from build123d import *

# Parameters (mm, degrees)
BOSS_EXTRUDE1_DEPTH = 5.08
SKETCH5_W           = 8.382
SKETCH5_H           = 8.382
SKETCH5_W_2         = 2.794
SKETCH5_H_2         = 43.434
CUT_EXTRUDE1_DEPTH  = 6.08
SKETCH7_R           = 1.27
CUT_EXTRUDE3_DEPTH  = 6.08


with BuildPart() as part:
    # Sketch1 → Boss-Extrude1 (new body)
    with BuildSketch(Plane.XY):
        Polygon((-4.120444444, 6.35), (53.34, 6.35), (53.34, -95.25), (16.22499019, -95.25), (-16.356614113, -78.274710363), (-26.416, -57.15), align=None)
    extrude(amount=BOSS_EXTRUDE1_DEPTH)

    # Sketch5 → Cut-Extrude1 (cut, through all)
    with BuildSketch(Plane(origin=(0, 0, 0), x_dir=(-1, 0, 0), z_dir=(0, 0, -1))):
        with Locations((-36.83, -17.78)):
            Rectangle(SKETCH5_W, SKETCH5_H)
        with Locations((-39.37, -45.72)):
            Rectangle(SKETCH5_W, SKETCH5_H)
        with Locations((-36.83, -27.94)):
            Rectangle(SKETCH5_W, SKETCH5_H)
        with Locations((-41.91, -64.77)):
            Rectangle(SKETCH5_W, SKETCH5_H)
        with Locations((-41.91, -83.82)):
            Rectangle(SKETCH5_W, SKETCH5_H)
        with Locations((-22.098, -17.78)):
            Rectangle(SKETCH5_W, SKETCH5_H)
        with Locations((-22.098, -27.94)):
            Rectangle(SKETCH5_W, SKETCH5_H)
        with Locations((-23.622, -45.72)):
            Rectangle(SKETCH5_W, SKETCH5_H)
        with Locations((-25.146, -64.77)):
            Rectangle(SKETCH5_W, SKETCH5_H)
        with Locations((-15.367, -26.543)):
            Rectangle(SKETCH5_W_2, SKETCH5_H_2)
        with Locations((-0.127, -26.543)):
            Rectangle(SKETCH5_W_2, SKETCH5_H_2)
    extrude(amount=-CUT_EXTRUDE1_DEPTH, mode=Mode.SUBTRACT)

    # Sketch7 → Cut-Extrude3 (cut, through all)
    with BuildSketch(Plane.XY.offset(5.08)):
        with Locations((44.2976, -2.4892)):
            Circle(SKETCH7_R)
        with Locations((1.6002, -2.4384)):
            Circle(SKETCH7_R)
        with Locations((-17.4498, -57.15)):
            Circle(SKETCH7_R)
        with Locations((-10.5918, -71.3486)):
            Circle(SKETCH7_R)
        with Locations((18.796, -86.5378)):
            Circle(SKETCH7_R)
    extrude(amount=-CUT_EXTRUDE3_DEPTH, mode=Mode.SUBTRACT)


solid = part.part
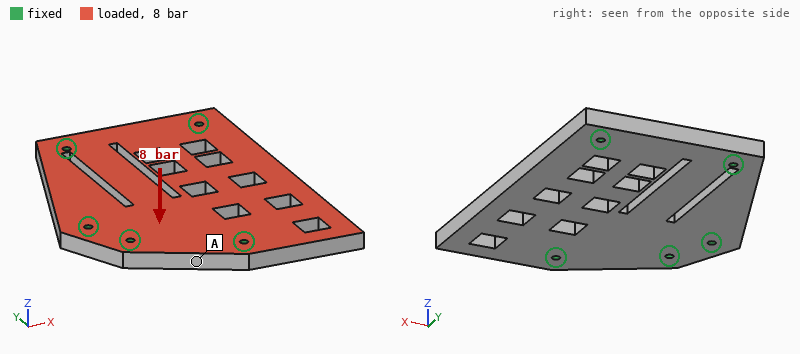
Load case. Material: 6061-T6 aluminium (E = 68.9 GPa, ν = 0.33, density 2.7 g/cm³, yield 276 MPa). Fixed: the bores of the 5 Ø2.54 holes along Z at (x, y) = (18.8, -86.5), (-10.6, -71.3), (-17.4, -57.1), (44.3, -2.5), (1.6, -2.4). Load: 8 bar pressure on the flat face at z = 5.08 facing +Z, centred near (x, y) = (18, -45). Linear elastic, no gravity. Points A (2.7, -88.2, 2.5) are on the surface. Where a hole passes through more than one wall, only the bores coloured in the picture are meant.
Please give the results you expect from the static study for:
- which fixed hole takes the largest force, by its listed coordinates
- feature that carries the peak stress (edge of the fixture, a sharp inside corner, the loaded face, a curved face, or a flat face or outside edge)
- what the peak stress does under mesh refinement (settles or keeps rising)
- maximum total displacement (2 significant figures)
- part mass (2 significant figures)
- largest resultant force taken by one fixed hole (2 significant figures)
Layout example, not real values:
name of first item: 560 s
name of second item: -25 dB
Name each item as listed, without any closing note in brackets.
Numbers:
which fixed hole takes the largest force, by its listed coordinates: (18.8, -86.5)
feature that carries the peak stress: edge of the fixture
what the peak stress does under mesh refinement: keeps rising
maximum total displacement: 0.38 mm
part mass: 81 g
largest resultant force taken by one fixed hole: 1.6 kN
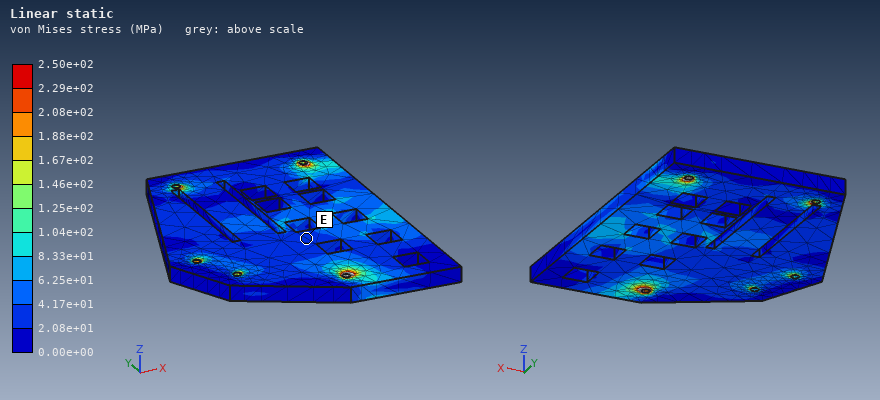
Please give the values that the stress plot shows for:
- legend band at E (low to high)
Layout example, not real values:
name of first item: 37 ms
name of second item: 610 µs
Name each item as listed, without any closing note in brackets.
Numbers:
legend band at E: 2.08e+01 to 4.17e+01 MPa
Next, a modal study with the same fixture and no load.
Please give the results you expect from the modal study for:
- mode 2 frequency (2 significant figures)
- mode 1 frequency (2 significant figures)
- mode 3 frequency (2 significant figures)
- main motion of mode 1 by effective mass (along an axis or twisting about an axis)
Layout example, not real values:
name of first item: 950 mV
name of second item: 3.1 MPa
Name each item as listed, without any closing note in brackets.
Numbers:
mode 2 frequency: 4200 Hz
mode 1 frequency: 2600 Hz
mode 3 frequency: 5800 Hz
main motion of mode 1 by effective mass: along Z
